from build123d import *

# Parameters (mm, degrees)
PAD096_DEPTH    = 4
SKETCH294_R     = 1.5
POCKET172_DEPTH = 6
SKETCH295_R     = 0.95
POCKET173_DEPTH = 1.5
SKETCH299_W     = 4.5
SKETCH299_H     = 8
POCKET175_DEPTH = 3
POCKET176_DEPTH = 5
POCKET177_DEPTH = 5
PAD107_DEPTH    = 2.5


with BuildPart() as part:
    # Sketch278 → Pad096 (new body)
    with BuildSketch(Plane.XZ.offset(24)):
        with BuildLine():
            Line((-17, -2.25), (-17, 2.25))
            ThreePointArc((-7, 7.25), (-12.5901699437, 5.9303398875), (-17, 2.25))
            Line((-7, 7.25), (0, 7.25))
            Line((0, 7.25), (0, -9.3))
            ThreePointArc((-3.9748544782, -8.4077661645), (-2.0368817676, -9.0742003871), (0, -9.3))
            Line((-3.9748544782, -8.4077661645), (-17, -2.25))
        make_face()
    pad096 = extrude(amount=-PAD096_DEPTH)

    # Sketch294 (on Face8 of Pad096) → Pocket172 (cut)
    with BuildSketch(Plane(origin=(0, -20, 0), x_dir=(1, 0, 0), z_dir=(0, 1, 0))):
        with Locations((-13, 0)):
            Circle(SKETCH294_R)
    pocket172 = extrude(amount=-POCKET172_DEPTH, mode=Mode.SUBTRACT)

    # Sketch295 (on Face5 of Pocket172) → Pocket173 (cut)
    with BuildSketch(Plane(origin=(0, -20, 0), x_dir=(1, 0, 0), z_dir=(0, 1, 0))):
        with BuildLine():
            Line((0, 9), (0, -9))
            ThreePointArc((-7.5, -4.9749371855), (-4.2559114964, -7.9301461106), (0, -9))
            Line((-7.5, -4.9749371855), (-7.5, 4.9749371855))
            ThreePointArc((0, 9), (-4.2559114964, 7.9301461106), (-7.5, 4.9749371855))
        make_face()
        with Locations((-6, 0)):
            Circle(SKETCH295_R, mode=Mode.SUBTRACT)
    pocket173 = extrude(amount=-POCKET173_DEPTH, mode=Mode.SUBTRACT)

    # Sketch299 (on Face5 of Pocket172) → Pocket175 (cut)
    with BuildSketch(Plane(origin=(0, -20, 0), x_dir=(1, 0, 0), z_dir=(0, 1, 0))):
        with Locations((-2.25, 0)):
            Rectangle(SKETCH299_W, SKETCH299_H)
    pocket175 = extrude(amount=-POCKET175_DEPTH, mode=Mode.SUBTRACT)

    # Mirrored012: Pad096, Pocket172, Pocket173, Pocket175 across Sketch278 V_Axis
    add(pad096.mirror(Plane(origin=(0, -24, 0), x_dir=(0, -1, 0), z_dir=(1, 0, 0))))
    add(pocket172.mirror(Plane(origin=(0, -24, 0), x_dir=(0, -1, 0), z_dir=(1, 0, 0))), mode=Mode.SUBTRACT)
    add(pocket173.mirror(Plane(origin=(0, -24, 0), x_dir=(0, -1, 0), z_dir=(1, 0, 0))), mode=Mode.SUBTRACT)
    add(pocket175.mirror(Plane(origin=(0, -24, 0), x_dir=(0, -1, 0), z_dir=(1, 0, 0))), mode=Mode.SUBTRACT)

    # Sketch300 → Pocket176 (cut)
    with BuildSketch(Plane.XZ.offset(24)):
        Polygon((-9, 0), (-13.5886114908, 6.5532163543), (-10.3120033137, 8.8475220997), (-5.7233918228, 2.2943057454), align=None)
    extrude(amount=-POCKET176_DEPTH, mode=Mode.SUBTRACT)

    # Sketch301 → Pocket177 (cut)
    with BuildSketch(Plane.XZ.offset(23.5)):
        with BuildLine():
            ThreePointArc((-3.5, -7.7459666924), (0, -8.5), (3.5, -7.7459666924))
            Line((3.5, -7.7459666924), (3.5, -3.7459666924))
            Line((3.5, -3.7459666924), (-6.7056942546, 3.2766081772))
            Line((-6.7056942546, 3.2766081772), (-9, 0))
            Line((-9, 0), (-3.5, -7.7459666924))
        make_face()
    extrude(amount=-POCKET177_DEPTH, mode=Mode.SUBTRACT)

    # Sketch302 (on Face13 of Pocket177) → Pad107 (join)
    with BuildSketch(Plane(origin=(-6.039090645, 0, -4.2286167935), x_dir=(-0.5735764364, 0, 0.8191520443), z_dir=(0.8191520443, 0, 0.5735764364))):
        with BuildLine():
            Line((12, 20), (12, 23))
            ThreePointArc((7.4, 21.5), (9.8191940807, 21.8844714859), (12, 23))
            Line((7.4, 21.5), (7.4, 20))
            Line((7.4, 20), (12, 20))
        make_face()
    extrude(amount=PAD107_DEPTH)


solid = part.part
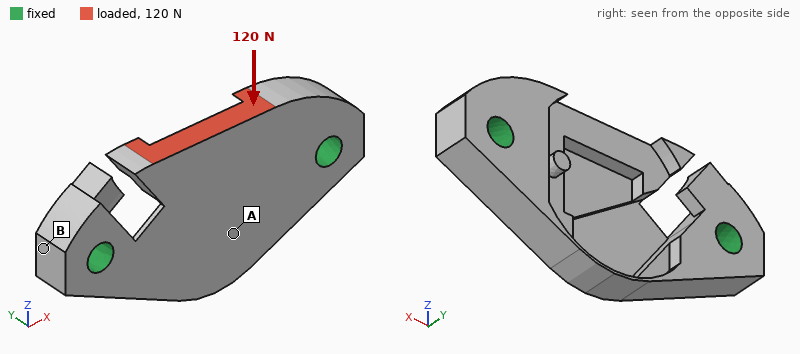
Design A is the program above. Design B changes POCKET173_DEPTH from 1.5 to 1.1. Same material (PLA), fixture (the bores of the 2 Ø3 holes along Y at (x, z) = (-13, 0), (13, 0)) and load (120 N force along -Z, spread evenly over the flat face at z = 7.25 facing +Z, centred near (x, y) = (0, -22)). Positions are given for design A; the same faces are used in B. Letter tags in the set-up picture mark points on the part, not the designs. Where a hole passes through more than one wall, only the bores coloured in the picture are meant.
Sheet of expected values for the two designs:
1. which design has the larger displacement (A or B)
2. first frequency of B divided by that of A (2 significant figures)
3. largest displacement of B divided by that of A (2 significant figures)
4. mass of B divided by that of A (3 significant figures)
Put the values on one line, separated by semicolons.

A; 1.1; 0.86; 1.04
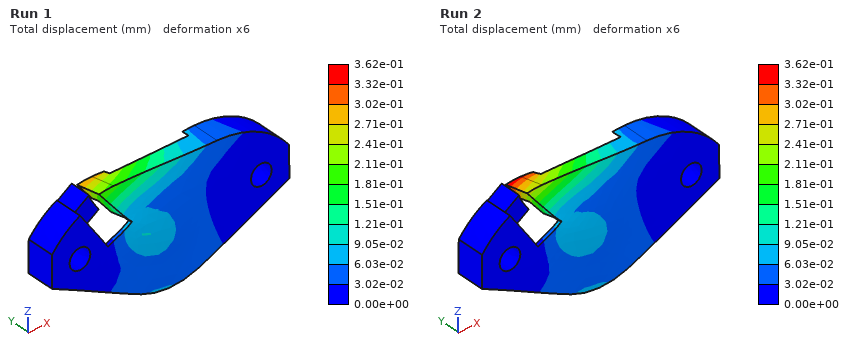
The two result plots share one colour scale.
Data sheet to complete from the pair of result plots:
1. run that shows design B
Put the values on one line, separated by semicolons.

Run 1
